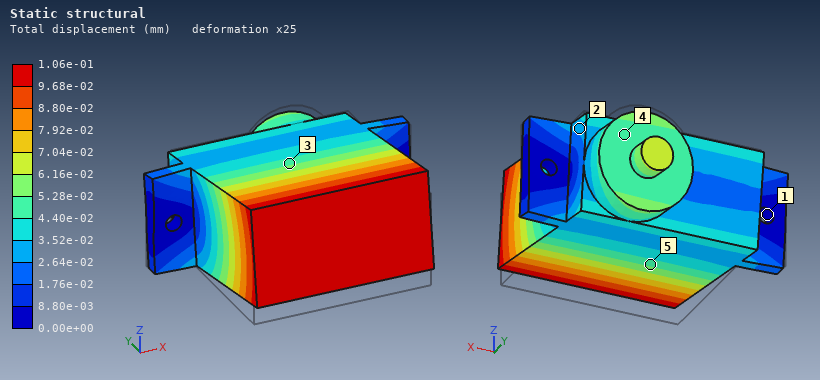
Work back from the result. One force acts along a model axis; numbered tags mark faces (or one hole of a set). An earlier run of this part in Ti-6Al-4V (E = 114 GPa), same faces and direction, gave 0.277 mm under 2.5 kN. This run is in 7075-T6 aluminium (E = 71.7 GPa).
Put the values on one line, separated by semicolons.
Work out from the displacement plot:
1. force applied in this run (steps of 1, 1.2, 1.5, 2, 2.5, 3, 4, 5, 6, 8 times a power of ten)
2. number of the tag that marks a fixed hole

600 N; 1
